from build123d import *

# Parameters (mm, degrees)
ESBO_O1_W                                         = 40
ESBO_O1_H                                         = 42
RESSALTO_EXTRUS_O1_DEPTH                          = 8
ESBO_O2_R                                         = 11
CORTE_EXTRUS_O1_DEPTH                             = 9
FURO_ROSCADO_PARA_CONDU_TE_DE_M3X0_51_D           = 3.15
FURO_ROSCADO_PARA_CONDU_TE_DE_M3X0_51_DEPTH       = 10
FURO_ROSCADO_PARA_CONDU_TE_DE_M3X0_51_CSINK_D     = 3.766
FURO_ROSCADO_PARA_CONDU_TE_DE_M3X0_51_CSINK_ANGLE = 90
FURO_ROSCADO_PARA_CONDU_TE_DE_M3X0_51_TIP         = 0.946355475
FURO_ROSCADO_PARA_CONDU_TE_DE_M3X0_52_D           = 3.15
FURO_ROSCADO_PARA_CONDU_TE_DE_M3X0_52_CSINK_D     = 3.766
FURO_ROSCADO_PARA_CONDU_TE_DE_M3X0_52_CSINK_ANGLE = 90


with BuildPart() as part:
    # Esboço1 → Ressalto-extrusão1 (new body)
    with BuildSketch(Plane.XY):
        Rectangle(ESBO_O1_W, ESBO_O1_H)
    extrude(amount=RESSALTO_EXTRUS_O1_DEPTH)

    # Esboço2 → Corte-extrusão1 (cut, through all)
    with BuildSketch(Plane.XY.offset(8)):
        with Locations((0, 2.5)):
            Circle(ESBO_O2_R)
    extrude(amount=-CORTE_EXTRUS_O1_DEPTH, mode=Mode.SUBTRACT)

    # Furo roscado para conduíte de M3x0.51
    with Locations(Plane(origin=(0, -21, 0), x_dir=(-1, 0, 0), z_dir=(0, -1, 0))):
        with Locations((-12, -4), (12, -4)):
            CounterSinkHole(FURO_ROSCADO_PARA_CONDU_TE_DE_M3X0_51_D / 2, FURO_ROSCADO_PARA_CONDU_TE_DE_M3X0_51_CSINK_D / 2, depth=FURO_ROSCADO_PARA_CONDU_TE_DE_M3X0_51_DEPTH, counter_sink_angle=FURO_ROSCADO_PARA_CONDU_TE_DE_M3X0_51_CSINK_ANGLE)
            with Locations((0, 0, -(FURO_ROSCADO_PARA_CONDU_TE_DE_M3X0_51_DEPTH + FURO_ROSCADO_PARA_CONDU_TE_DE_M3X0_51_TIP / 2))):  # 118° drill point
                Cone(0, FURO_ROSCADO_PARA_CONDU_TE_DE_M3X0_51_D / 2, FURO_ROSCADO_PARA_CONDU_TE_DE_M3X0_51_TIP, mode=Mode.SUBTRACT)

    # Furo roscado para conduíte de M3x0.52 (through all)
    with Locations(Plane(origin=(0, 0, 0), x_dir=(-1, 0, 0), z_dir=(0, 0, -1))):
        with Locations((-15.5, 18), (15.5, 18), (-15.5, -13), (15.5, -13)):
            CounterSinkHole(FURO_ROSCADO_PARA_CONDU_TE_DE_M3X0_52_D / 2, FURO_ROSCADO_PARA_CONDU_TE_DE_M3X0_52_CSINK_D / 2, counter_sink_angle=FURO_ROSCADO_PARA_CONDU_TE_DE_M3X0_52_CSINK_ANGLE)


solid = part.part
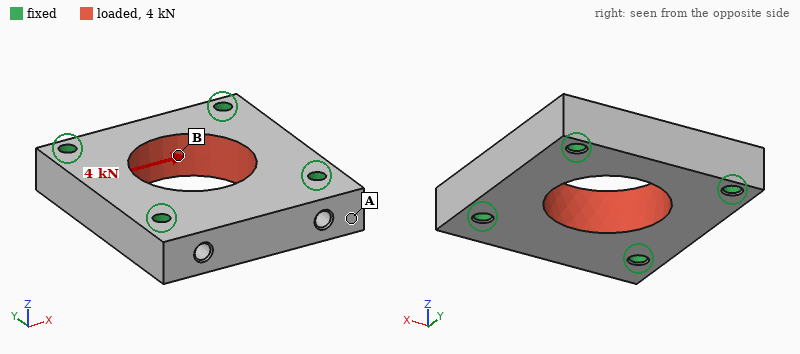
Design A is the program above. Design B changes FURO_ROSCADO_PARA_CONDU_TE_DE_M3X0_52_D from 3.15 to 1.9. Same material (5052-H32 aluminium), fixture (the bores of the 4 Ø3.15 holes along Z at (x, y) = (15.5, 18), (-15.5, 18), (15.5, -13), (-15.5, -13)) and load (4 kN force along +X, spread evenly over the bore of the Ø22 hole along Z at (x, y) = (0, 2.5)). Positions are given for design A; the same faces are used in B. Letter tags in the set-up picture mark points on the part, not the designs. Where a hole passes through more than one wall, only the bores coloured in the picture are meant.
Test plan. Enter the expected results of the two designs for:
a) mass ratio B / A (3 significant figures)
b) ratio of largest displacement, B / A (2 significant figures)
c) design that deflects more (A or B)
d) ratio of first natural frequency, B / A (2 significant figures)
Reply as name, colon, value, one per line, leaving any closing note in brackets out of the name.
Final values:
mass ratio B / A: 1.01
ratio of largest displacement, B / A: 1.1
design that deflects more: B
ratio of first natural frequency, B / A: 0.87
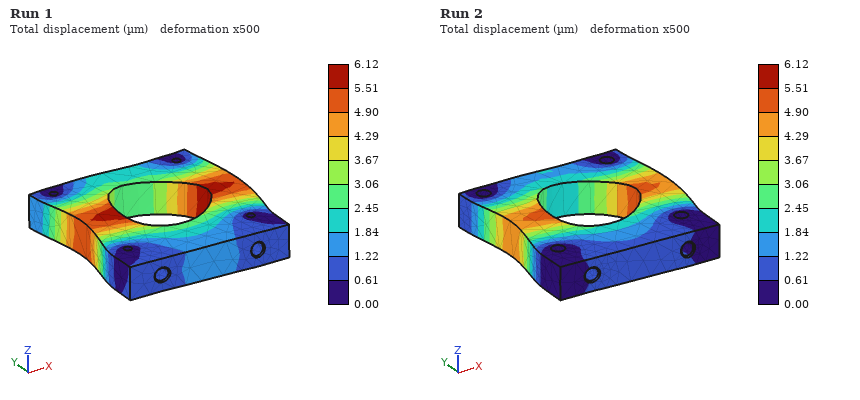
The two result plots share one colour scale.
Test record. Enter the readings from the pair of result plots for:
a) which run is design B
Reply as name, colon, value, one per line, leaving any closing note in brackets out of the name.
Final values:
which run is design B: Run 1
